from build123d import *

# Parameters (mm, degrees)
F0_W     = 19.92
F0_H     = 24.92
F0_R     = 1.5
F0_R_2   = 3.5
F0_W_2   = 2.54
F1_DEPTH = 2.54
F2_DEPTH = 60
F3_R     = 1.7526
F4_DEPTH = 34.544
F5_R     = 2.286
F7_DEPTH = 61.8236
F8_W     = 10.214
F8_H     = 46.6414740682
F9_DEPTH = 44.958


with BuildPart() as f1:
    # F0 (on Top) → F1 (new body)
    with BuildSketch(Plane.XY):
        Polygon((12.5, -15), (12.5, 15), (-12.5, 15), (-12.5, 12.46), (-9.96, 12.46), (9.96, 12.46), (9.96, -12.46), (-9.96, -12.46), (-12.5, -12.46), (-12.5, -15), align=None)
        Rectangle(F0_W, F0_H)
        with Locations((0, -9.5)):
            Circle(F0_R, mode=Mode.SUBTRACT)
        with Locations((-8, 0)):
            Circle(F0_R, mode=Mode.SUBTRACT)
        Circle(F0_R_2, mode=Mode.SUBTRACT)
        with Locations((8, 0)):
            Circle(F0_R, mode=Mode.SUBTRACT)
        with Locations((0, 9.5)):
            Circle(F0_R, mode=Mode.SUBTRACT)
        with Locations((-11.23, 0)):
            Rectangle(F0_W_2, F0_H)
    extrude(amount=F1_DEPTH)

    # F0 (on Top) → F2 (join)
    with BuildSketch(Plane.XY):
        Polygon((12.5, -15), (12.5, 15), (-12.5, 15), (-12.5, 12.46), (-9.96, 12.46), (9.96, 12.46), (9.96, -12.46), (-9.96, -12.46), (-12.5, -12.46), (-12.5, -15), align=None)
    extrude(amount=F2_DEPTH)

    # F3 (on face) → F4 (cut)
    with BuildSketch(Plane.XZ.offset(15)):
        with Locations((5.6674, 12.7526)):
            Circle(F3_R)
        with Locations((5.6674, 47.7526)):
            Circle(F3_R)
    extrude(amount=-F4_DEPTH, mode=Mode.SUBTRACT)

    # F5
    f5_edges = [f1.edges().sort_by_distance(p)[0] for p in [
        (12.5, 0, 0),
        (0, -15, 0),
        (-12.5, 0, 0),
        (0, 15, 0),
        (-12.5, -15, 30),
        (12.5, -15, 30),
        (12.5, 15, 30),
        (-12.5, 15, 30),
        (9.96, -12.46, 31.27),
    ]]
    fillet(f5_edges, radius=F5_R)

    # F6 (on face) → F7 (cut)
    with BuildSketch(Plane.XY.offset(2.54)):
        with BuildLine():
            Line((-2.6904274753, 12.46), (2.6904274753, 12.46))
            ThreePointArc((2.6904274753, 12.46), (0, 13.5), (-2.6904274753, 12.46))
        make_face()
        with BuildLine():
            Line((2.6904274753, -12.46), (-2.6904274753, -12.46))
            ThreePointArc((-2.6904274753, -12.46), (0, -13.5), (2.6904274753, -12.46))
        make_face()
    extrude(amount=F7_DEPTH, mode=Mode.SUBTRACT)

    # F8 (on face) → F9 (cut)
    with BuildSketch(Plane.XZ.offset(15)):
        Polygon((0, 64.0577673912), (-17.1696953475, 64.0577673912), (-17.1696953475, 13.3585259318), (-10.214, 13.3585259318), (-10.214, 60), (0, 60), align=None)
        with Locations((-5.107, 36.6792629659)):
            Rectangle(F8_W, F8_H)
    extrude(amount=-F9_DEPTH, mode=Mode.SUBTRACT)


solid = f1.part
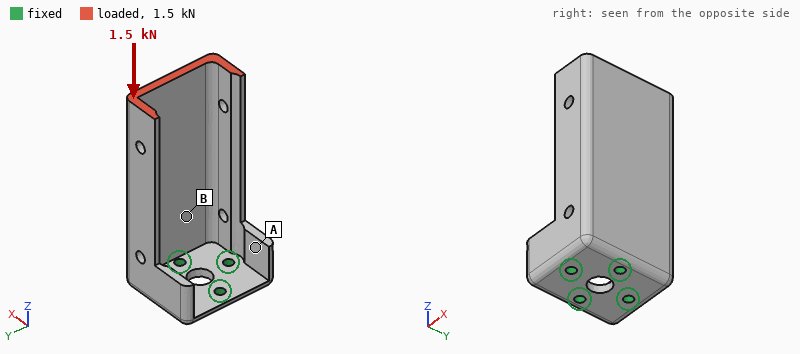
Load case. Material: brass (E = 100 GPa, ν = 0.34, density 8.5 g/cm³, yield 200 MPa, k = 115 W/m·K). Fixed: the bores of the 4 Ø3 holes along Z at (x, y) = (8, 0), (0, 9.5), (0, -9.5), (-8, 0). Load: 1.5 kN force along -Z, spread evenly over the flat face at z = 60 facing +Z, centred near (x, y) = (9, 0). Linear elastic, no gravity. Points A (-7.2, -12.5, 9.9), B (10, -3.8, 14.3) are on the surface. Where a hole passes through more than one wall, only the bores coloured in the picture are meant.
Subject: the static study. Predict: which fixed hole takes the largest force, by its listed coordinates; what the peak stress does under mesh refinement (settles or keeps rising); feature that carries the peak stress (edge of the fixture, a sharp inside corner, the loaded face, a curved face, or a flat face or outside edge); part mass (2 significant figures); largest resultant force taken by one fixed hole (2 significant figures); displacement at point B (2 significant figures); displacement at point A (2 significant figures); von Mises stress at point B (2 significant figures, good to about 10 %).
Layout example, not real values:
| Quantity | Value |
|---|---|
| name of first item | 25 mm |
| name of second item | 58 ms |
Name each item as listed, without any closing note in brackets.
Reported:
| Quantity | Value |
|---|---|
| which fixed hole takes the largest force, by its listed coordinates | (8, 0) |
| what the peak stress does under mesh refinement | keeps rising |
| feature that carries the peak stress | edge of the fixture |
| part mass | 78 g |
| largest resultant force taken by one fixed hole | 1.1 kN |
| displacement at point B | 15 µm |
| displacement at point A | 7.2 µm |
| von Mises stress at point B | 22 MPa |
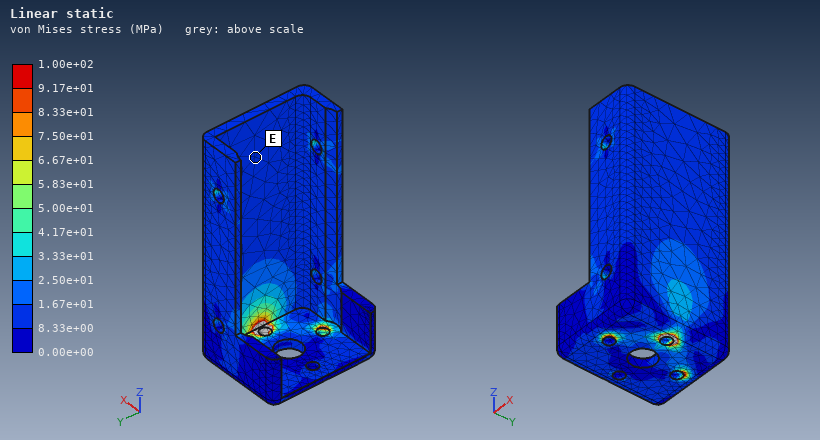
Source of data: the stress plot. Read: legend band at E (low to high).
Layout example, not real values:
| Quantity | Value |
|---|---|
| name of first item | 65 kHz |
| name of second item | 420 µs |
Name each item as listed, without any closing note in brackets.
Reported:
| Quantity | Value |
|---|---|
| legend band at E | 8.33e+00 to 1.67e+01 MPa |
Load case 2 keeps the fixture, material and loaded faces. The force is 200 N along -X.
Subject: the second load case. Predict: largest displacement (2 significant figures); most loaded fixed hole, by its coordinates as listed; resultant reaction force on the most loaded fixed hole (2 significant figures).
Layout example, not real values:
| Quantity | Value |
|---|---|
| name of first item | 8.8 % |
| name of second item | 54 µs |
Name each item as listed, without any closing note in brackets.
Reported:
| Quantity | Value |
|---|---|
| largest displacement | 0.17 mm |
| most loaded fixed hole, by its coordinates as listed | (8, 0) |
| resultant reaction force on the most loaded fixed hole | 910 N |
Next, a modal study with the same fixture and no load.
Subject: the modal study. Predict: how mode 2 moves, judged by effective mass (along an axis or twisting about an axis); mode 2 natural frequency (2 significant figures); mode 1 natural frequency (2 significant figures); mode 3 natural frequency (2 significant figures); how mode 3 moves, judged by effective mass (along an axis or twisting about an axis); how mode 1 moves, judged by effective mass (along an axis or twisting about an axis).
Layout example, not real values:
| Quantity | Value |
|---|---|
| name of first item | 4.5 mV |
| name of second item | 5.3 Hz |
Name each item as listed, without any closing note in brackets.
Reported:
| Quantity | Value |
|---|---|
| how mode 2 moves, judged by effective mass | along X |
| mode 2 natural frequency | 1400 Hz |
| mode 1 natural frequency | 1100 Hz |
| mode 3 natural frequency | 3200 Hz |
| how mode 3 moves, judged by effective mass | along Y |
| how mode 1 moves, judged by effective mass | along Y |
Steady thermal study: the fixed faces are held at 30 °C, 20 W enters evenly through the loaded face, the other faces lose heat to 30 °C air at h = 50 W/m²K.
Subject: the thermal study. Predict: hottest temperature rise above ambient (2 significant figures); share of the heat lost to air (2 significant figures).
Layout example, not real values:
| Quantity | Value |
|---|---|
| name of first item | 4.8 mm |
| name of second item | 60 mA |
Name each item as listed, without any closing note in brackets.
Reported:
| Quantity | Value |
|---|---|
| hottest temperature rise above ambient | 64 K |
| share of the heat lost to air | 46 % |
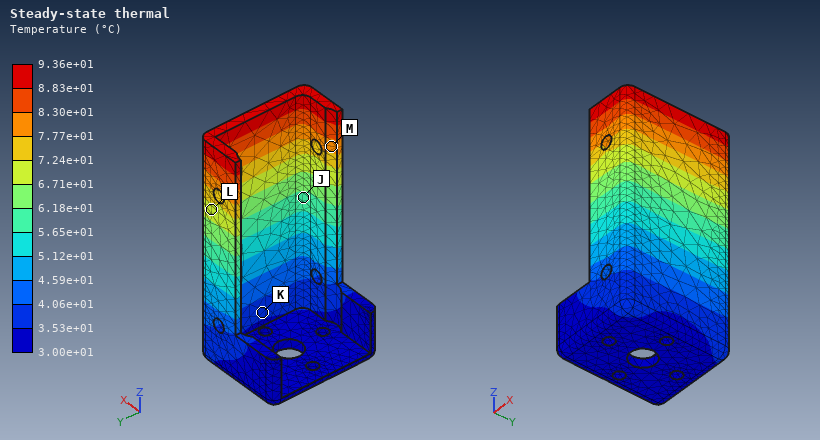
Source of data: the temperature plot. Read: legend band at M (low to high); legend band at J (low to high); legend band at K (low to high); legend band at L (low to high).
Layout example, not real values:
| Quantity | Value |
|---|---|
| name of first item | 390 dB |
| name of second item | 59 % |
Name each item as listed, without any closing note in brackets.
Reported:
| Quantity | Value |
|---|---|
| legend band at M | 7.77e+01 to 8.30e+01 °C |
| legend band at J | 5.65e+01 to 6.18e+01 °C |
| legend band at K | 3.53e+01 to 4.06e+01 °C |
| legend band at L | 6.71e+01 to 7.24e+01 °C |
